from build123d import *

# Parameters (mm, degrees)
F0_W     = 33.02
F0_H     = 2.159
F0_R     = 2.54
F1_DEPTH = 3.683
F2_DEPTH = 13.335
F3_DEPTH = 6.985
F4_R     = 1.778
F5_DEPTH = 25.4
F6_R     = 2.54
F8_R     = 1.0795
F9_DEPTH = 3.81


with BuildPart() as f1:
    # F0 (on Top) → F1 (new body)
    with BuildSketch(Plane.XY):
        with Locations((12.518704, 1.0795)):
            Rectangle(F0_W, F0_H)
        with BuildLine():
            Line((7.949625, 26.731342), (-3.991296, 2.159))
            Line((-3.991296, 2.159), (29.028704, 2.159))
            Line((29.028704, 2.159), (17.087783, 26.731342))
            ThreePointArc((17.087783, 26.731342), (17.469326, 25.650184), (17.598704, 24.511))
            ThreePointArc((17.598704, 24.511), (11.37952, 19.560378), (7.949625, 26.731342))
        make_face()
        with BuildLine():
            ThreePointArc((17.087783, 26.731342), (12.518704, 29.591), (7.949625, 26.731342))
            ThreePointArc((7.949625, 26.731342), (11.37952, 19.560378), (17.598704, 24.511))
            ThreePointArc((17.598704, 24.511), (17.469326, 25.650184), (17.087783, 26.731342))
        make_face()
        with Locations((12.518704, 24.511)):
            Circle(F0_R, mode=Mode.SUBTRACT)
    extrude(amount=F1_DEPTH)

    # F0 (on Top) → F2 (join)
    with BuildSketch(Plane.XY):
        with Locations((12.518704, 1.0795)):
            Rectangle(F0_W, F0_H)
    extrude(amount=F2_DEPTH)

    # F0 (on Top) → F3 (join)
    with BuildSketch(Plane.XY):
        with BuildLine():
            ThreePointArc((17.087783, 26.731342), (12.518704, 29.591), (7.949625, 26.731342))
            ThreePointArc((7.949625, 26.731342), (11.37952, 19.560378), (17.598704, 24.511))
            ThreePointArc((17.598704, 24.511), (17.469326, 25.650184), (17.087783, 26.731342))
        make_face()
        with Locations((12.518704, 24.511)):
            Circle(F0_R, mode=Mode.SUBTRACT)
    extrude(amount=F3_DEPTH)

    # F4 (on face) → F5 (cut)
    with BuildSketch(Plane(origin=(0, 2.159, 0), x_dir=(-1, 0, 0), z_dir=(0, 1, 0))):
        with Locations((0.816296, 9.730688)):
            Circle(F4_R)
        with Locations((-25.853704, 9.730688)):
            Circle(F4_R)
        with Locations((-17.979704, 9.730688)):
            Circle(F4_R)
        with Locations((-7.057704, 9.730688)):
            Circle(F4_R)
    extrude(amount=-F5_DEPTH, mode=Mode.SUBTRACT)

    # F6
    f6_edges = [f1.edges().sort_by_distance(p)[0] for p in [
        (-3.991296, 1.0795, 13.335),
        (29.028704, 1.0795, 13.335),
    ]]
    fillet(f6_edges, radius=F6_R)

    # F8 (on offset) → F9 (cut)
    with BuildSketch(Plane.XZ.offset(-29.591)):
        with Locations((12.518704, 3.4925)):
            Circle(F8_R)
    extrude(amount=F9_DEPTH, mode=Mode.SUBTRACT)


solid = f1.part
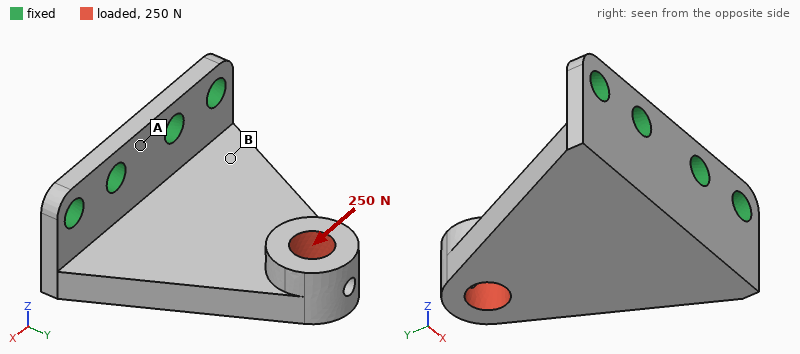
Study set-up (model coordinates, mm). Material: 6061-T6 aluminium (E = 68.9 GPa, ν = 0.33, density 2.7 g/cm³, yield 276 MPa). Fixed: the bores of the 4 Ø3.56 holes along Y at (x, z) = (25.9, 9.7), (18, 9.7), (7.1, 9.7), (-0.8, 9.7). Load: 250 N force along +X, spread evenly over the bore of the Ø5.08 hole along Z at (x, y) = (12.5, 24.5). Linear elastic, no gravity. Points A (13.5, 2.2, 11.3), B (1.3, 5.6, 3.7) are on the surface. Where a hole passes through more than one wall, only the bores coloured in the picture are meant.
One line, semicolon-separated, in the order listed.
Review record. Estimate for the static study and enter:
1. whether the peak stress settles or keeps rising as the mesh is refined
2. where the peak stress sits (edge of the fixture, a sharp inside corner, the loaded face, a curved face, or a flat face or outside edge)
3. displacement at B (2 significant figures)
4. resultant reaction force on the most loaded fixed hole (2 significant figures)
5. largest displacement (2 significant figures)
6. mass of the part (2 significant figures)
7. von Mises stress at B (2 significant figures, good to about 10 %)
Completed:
keeps rising; edge of the fixture; 16 µm; 200 N; 55 µm; 8.0 g; 32 MPa
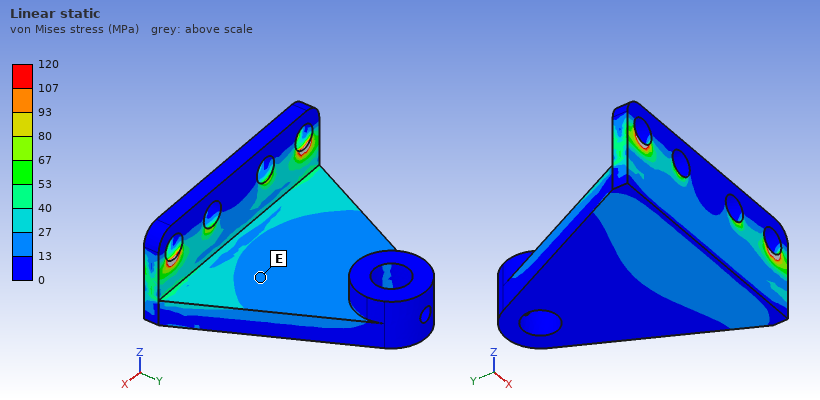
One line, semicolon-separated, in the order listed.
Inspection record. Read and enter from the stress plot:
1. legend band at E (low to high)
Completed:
13 to 27 MPa
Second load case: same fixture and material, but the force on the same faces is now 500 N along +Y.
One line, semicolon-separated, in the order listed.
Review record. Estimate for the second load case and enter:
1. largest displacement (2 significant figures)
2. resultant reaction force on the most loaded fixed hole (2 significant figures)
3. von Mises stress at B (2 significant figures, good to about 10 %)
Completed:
52 µm; 140 N; 17 MPa
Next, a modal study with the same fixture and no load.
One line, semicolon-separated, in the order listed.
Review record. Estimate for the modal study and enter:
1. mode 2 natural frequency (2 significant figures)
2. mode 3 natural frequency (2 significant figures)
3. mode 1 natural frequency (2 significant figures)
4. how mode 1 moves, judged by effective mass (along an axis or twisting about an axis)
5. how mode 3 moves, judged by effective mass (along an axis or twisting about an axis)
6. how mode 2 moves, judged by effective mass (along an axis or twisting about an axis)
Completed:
7900 Hz; 12 kHz; 2400 Hz; along Z; along Y; along X
